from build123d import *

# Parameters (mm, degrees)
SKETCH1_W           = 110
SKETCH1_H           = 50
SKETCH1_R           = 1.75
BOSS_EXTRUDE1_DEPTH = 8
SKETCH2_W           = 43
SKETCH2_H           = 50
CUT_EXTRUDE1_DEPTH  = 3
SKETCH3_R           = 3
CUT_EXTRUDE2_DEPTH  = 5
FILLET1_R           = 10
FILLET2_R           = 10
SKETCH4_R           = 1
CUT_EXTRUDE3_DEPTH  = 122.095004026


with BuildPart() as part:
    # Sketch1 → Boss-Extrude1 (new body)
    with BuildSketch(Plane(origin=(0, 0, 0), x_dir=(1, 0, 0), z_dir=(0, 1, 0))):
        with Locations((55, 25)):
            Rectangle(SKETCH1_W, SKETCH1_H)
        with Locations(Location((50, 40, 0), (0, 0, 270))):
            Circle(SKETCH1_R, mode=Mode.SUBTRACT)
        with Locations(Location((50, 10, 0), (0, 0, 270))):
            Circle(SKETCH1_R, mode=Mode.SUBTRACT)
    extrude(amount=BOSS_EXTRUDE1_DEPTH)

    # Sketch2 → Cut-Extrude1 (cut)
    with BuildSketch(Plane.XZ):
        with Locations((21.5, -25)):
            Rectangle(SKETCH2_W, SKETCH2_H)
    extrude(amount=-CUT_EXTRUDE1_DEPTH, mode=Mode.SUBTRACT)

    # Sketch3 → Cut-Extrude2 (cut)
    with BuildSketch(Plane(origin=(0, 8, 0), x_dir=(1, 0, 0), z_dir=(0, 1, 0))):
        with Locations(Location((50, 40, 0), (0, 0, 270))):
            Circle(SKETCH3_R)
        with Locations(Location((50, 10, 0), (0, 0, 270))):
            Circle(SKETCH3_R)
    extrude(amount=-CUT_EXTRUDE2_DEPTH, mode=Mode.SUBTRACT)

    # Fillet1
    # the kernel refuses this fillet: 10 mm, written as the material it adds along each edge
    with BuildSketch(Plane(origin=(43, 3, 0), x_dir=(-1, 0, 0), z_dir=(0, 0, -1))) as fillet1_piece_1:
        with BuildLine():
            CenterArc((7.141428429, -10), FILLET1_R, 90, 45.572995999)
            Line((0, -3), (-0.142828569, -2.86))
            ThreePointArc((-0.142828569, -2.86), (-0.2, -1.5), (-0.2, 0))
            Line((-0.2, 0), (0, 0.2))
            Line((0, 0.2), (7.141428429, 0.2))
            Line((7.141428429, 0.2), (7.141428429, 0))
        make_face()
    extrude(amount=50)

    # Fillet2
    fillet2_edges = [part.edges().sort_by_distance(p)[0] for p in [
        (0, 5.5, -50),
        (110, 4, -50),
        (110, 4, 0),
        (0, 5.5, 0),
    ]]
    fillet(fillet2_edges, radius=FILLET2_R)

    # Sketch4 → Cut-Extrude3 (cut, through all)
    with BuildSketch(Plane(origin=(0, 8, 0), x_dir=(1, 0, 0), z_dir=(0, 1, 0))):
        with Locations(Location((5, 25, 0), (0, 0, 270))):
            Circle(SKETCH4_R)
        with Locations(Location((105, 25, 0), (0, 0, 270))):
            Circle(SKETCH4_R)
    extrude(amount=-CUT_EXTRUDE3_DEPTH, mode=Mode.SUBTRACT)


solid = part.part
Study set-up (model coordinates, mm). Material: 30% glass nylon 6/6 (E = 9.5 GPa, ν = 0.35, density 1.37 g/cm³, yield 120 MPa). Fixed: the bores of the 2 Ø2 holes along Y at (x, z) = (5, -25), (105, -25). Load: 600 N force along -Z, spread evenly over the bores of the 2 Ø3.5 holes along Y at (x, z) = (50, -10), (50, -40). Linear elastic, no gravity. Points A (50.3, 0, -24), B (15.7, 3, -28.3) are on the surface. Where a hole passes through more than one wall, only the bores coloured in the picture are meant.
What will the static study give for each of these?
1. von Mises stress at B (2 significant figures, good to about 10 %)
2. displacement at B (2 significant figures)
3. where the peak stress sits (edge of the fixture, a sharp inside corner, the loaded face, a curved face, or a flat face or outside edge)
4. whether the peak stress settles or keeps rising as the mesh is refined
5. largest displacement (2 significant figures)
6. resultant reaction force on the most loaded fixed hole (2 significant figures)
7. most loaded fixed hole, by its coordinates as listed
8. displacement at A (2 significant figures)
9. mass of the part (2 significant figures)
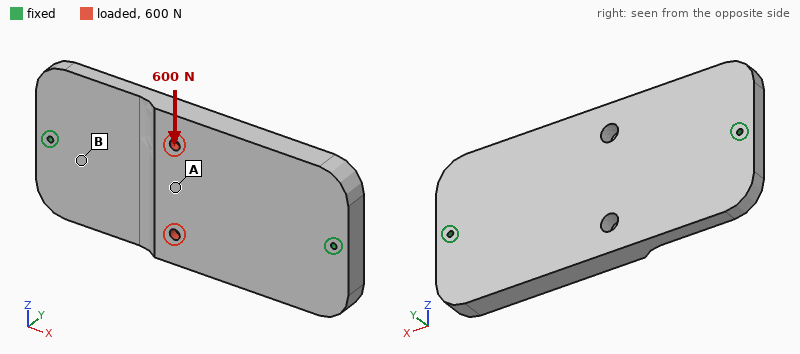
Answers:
5.7 MPa
0.020 mm
edge of the fixture
keeps rising
0.12 mm
330 N
(5, -25)
0.055 mm
51 g
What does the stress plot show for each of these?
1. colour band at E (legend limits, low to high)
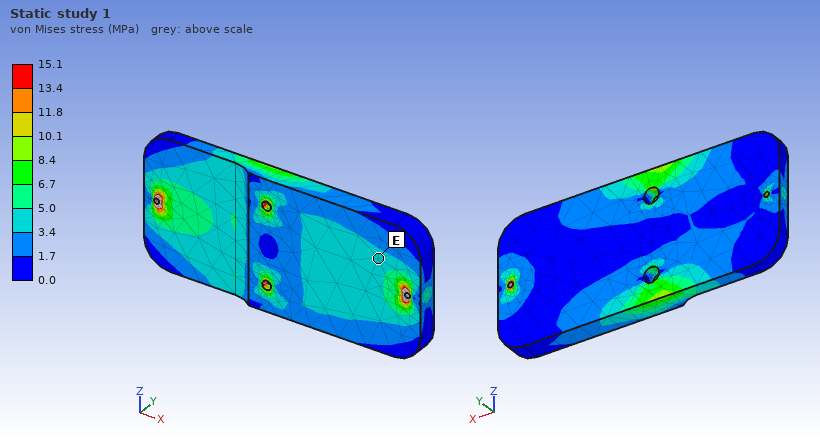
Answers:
3.4 to 5.0 MPa
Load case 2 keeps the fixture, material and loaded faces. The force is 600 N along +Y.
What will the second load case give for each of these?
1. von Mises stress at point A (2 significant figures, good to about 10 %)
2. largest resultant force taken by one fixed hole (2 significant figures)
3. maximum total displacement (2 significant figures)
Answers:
18 MPa
310 N
0.53 mm
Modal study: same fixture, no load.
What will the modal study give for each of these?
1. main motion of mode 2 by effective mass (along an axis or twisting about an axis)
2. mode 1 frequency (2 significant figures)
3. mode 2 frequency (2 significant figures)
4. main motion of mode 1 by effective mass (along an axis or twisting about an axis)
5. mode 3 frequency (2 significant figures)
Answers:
twisting about X
1200 Hz
1400 Hz
along Y
3100 Hz
